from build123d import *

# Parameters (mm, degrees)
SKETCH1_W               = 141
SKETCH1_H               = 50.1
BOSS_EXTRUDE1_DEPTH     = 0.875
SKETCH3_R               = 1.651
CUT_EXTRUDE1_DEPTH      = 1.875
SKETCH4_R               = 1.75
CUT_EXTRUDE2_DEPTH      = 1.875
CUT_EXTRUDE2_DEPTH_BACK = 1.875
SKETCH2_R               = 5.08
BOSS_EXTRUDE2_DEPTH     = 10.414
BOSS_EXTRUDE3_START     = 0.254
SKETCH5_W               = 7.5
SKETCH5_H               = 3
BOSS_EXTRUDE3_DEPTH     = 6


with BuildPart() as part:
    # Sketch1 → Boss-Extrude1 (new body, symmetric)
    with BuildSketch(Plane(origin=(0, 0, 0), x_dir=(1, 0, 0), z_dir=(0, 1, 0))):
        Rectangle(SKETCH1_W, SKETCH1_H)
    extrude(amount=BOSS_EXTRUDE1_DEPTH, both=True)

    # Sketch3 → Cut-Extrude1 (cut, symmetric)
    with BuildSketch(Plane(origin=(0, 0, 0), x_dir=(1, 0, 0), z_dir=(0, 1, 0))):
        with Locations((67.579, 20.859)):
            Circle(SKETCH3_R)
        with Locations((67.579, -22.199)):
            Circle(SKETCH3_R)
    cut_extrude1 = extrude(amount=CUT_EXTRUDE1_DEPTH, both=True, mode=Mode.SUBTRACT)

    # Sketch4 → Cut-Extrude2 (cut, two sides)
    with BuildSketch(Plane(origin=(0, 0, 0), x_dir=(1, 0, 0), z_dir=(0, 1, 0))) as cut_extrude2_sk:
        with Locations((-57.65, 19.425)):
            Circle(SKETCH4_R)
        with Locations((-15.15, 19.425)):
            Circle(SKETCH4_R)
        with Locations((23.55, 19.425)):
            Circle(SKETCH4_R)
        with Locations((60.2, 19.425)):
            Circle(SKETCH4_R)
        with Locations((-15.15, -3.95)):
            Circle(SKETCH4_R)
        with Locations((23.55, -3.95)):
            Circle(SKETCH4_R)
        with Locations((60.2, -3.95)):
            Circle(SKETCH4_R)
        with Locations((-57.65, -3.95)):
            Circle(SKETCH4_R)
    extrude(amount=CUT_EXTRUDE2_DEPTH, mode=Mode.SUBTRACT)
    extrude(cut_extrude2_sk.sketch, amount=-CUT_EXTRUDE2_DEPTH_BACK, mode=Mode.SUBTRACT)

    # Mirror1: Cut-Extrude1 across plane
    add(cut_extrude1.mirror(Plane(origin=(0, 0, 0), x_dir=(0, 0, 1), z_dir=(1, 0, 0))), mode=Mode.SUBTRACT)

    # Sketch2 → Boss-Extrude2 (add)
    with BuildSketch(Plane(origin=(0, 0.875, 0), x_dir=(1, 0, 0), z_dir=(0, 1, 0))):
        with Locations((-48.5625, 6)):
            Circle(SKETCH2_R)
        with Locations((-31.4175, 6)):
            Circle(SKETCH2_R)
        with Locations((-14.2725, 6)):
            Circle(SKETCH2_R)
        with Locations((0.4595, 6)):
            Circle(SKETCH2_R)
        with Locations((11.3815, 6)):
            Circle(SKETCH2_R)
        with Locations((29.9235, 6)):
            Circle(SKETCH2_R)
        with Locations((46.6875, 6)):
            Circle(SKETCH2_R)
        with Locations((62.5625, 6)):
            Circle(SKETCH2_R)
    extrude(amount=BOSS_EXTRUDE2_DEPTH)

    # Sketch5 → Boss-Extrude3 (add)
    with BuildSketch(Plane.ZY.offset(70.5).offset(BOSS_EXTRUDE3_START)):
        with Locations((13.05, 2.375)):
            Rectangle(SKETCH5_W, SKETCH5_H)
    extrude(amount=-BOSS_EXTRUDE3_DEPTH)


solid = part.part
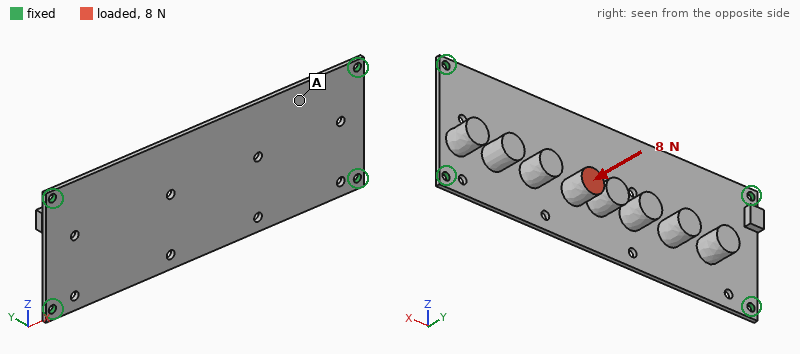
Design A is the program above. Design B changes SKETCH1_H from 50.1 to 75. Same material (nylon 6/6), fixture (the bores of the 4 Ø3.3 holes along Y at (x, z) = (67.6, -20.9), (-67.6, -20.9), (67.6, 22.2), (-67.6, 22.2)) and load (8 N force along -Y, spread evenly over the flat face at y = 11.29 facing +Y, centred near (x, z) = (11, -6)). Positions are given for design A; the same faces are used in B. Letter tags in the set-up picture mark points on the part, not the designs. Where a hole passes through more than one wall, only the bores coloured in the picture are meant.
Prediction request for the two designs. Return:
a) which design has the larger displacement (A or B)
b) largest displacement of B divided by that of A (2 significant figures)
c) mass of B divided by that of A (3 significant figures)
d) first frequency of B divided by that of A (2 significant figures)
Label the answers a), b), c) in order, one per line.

a) A
b) 0.70
c) 1.32
d) 1.1
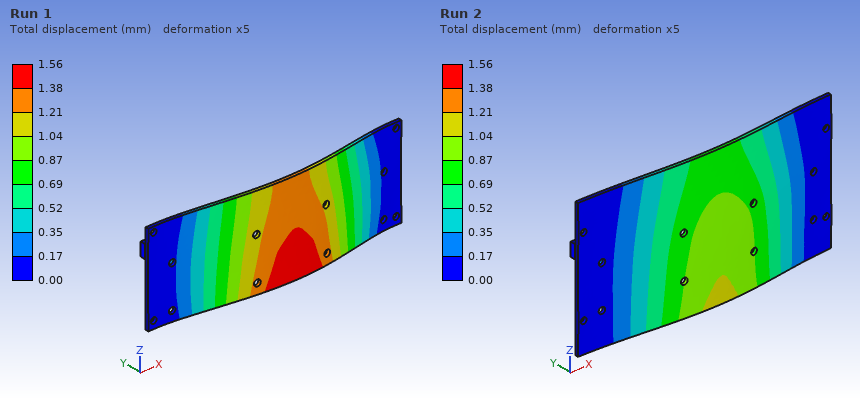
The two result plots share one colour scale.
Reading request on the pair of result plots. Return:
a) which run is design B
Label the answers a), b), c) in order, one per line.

a) Run 2
